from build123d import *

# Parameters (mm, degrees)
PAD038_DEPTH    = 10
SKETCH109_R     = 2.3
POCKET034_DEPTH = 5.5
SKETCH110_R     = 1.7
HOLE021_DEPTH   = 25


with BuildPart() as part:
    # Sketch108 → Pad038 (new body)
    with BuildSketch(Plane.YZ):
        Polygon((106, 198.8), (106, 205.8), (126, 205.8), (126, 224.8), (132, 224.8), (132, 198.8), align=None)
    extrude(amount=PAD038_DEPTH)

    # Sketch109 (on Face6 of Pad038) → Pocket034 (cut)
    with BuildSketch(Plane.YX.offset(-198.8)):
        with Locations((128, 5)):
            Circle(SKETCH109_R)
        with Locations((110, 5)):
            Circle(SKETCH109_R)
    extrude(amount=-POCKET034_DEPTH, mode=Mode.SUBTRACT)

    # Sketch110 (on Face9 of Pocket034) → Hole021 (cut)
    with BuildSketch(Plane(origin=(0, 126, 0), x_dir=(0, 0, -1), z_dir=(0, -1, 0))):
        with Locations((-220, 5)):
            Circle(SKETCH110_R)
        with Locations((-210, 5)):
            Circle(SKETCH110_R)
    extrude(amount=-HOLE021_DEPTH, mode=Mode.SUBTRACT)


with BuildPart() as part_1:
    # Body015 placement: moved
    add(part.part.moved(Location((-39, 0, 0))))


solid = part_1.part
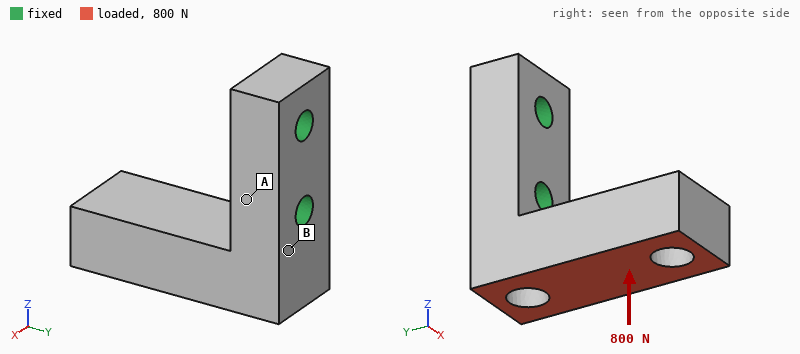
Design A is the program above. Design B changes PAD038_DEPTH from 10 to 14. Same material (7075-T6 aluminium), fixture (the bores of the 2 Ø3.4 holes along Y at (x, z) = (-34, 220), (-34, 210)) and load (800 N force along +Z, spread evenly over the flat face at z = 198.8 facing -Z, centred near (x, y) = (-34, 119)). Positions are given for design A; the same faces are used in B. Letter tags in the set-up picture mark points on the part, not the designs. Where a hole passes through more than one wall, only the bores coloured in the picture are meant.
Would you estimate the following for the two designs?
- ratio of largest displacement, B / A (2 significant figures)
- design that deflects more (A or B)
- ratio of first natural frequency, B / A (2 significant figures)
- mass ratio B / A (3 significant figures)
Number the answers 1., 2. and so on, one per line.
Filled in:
1. 0.75
2. A
3. 0.96
4. 1.44
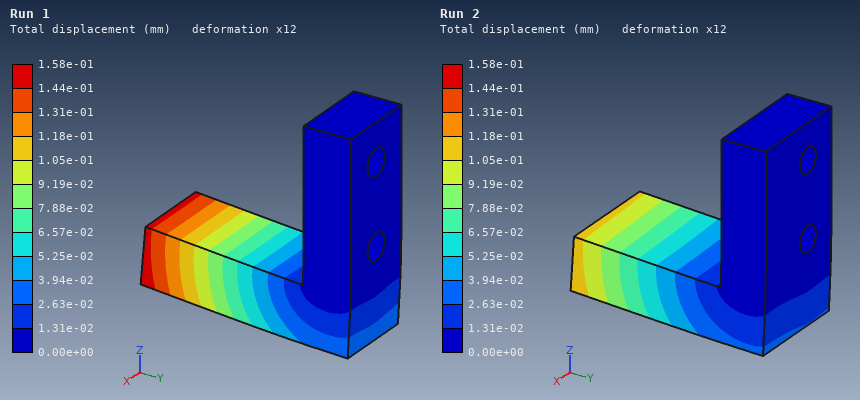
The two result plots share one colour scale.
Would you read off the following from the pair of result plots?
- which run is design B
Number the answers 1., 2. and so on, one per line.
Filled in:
1. Run 2
